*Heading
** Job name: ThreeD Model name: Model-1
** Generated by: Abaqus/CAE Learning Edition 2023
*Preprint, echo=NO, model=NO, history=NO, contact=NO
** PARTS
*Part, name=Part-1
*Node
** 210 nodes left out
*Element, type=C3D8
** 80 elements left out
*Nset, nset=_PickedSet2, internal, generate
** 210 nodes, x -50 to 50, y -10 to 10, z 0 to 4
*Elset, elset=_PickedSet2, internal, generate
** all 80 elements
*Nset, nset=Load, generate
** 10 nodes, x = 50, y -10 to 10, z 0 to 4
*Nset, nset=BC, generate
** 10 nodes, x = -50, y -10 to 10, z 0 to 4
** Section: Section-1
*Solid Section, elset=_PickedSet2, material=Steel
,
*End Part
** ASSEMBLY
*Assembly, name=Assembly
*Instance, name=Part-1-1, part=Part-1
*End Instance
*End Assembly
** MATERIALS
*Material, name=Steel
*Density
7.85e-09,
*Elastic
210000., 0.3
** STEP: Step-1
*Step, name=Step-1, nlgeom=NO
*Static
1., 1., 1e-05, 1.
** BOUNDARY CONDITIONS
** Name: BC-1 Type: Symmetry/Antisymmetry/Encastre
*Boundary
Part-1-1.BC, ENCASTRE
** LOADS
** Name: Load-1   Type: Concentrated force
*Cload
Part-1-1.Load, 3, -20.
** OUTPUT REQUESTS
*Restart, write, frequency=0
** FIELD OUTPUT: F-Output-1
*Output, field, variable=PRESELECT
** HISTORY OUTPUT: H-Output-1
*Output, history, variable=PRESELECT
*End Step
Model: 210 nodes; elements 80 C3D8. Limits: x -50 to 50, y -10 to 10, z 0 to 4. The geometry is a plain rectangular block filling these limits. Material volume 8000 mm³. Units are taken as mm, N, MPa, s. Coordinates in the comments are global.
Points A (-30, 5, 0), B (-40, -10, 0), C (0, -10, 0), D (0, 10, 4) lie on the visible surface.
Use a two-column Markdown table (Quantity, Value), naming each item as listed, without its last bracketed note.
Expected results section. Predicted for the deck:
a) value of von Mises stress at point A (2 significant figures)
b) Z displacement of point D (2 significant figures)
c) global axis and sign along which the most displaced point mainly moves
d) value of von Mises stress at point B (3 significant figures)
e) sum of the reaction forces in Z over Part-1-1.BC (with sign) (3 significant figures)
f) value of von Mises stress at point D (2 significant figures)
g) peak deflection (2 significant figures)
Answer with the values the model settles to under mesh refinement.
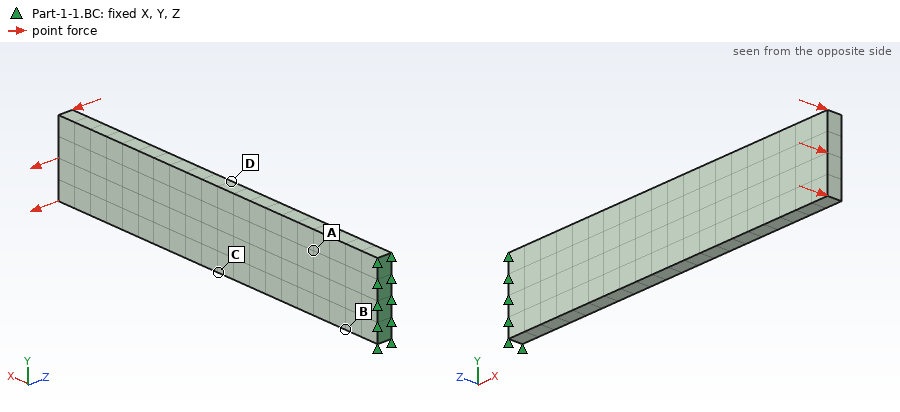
| Quantity | Value |
|---|---|
| value of von Mises stress at point A | 300 MPa |
| Z displacement of point D | -0.89 mm |
| global axis and sign along which the most displaced point mainly moves | -Z |
| value of von Mises stress at point B | 335 MPa |
| sum of the reaction forces in Z over Part-1-1.BC (with sign) | 200 N |
| value of von Mises stress at point D | 190 MPa |
| peak deflection | 2.9 mm |
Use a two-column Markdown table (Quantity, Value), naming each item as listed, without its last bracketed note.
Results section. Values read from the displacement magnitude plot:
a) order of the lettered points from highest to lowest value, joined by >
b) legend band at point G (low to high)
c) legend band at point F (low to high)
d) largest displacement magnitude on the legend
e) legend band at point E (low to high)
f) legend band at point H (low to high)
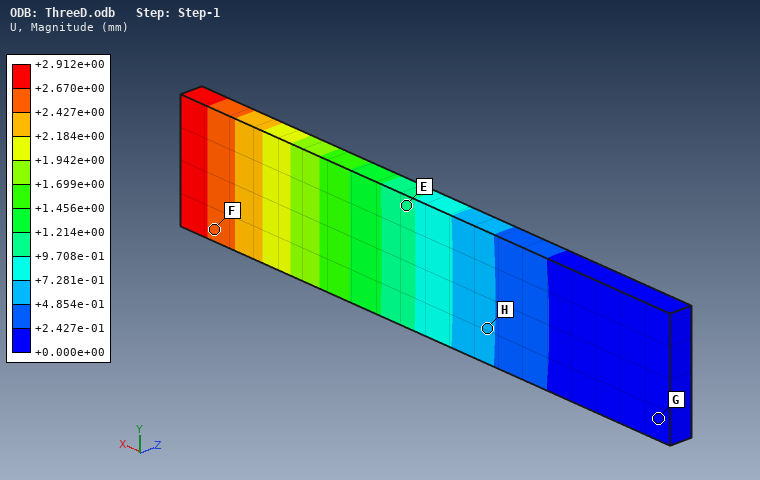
| Quantity | Value |
|---|---|
| order of the lettered points from highest to lowest value, joined by > | F > E > H > G |
| legend band at point G | +0.000e+00 to +2.427e-01 mm |
| legend band at point F | +2.427e+00 to +2.670e+00 mm |
| largest displacement magnitude on the legend | +2.912e+00 mm |
| legend band at point E | +9.708e-01 to +1.214e+00 mm |
| legend band at point H | +4.854e-01 to +7.281e-01 mm |
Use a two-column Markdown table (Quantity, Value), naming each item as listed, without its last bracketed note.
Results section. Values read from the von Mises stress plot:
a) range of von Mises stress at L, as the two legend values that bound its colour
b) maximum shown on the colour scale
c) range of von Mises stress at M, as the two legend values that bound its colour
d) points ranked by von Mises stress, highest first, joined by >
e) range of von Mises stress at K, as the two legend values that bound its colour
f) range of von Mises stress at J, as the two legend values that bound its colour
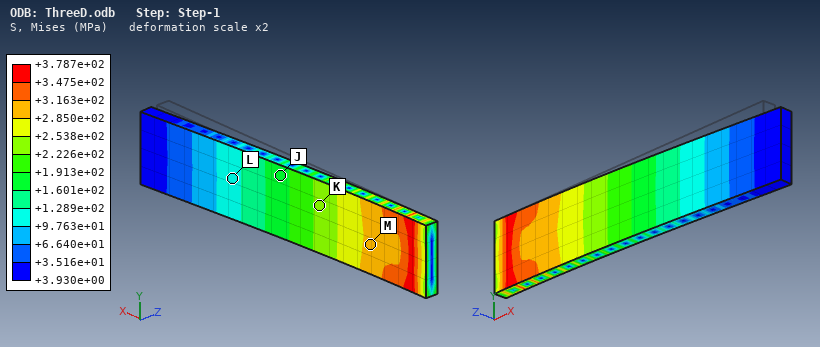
| Quantity | Value |
|---|---|
| range of von Mises stress at L, as the two legend values that bound its colour | +9.763e+01 to +1.289e+02 MPa |
| maximum shown on the colour scale | +3.787e+02 MPa |
| range of von Mises stress at M, as the two legend values that bound its colour | +2.850e+02 to +3.163e+02 MPa |
| points ranked by von Mises stress, highest first, joined by > | M > K > J > L |
| range of von Mises stress at K, as the two legend values that bound its colour | +2.226e+02 to +2.538e+02 MPa |
| range of von Mises stress at J, as the two legend values that bound its colour | +1.601e+02 to +1.913e+02 MPa |
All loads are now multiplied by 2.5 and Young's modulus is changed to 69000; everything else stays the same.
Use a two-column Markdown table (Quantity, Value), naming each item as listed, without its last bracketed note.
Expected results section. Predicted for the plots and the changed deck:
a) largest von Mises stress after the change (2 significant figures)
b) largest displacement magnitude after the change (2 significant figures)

| Quantity | Value |
|---|---|
| largest von Mises stress after the change | 950 MPa |
| largest displacement magnitude after the change | 22 mm |
